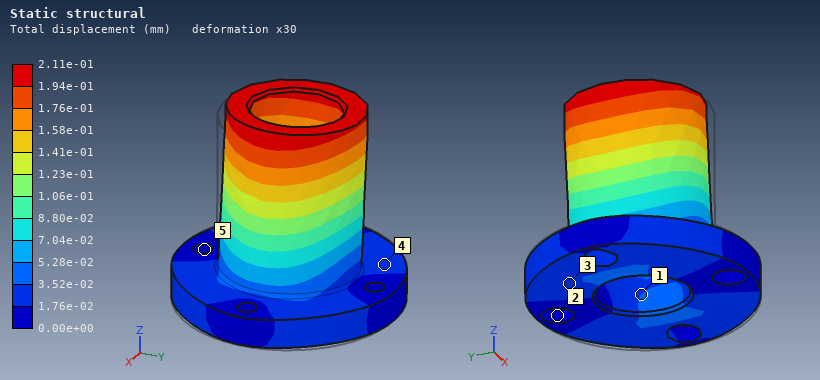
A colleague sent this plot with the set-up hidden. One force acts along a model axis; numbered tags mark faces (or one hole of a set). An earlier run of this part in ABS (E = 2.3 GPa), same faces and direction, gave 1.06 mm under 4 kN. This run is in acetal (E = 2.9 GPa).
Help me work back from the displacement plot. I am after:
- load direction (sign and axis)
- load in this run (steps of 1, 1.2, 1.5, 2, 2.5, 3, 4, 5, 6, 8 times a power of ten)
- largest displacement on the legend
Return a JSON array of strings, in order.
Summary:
["-X", "1 kN", "2.11e-01 mm"]
